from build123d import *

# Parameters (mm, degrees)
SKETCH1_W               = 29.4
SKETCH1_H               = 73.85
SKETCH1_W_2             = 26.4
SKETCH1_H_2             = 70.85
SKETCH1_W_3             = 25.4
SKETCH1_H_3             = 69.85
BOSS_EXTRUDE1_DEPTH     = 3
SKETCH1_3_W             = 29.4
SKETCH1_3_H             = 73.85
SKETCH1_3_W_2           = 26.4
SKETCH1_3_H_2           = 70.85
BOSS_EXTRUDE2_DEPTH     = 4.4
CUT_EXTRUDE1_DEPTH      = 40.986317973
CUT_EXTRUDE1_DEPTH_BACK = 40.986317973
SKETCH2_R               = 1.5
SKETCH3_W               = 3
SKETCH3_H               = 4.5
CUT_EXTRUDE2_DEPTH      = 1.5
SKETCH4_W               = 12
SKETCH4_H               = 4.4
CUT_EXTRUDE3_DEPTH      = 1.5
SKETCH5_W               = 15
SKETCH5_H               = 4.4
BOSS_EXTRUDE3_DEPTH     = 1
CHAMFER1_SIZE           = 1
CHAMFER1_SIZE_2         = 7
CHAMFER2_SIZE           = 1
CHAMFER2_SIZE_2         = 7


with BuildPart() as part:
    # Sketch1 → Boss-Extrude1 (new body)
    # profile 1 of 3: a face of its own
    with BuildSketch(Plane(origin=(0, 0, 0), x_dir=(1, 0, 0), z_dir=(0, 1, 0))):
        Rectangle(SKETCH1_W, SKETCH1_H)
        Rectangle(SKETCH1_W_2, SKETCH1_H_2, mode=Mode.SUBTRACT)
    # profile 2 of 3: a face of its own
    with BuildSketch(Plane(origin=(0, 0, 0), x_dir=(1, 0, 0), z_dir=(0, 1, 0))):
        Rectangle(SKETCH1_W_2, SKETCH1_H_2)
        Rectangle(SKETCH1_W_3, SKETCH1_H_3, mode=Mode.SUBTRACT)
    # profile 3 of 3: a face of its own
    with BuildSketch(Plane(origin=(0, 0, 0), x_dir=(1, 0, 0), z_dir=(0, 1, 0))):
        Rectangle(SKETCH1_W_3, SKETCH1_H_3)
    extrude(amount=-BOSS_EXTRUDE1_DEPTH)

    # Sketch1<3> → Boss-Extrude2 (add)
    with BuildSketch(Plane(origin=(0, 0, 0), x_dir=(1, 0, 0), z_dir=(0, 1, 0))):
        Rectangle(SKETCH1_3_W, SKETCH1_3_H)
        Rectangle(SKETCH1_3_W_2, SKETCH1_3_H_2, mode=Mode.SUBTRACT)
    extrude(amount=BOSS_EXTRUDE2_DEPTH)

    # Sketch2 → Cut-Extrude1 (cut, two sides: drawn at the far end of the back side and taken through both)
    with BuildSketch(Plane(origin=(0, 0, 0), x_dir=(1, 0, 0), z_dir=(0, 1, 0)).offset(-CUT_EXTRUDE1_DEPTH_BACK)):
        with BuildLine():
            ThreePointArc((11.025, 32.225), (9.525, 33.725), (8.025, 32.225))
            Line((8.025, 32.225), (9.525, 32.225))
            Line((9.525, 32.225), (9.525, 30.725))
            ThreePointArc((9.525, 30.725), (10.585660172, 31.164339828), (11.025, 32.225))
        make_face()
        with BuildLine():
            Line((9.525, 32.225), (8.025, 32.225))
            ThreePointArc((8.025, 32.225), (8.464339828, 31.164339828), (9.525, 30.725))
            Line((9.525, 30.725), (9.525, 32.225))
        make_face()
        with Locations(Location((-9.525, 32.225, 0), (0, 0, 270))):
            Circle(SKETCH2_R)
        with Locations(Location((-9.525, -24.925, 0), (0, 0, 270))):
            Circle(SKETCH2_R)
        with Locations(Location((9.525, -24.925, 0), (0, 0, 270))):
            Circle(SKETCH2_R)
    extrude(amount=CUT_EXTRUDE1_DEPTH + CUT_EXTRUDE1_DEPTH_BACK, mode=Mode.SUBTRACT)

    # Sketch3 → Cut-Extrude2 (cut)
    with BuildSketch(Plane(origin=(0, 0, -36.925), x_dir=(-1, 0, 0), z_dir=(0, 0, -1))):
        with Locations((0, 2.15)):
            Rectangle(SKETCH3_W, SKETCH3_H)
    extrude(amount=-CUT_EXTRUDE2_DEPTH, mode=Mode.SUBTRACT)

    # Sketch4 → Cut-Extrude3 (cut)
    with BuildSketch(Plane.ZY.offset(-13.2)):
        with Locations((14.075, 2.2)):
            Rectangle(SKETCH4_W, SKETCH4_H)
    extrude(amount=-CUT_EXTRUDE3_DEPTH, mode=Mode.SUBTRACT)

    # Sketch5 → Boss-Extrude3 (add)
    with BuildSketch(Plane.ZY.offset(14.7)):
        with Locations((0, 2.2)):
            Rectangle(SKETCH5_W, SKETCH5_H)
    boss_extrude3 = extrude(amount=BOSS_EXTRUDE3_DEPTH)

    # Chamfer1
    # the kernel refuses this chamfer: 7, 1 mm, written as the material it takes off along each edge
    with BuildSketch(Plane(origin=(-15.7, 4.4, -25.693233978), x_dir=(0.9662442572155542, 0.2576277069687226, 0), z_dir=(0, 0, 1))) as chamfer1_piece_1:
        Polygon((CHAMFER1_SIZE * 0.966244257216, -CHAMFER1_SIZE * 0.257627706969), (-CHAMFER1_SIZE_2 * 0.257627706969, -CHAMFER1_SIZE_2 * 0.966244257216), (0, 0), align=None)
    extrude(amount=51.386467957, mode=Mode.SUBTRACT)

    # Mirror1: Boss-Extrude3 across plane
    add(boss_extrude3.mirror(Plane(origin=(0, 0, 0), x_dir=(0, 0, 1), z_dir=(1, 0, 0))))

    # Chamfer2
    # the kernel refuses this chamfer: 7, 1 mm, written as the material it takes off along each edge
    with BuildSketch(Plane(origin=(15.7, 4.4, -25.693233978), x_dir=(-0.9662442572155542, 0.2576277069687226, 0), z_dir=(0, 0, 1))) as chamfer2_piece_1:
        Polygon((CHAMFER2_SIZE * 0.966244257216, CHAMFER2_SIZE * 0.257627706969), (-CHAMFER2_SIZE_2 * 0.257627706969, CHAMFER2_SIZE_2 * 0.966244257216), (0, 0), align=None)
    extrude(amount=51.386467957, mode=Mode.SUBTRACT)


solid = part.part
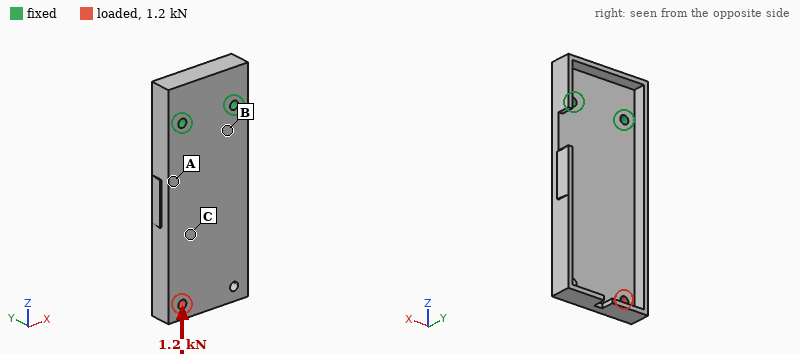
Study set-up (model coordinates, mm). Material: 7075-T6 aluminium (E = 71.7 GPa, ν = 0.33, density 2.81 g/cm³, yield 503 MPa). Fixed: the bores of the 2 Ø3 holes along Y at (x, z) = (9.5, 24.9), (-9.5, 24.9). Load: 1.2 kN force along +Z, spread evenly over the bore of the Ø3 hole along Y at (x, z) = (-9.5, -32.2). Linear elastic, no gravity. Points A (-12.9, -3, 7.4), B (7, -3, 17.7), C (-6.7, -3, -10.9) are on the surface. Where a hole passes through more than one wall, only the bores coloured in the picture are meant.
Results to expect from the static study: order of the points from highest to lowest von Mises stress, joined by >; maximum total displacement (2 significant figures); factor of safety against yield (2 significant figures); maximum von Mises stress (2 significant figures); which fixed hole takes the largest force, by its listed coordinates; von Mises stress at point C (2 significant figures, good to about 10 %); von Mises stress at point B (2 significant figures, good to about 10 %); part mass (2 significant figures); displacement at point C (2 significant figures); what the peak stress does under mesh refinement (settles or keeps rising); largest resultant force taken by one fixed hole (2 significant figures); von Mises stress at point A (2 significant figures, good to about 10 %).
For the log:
A > C > B
0.11 mm
5.1
98 MPa
(-9.5, 24.9)
28 MPa
8.6 MPa
22 g
0.040 mm
settles
1.2 kN
39 MPa
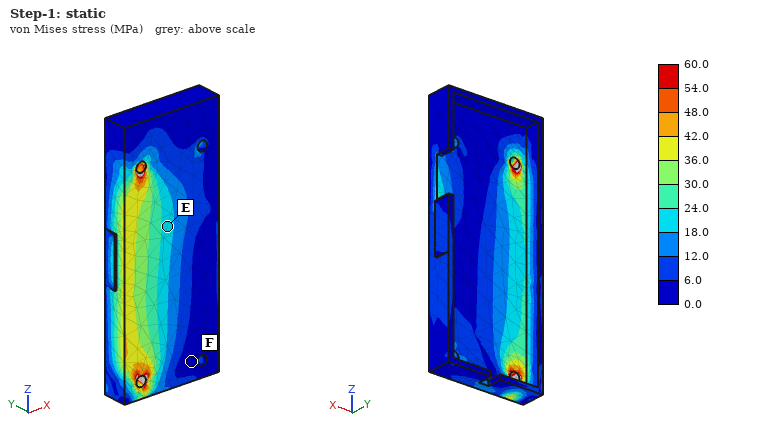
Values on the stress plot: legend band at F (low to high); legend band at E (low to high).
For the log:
0.0 to 6.0 MPa
18.0 to 24.0 MPa
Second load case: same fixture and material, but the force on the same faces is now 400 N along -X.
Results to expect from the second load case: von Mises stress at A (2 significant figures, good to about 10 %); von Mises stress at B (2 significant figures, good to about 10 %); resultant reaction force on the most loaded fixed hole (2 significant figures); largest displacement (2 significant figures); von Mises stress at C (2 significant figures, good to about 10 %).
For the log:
33 MPa
21 MPa
1.1 kN
0.10 mm
10 MPa
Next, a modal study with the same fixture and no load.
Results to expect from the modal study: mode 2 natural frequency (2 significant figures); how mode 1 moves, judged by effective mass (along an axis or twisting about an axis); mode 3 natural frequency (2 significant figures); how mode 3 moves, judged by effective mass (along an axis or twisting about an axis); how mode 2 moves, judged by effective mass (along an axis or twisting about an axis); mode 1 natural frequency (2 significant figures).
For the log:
2500 Hz
along Y
4900 Hz
along X
twisting about Z
780 Hz
